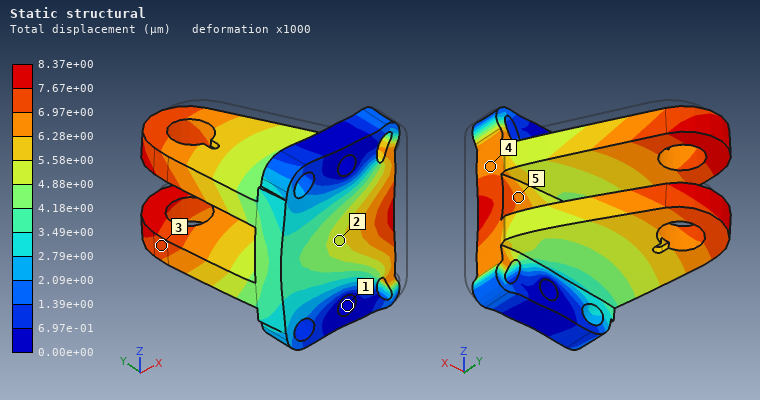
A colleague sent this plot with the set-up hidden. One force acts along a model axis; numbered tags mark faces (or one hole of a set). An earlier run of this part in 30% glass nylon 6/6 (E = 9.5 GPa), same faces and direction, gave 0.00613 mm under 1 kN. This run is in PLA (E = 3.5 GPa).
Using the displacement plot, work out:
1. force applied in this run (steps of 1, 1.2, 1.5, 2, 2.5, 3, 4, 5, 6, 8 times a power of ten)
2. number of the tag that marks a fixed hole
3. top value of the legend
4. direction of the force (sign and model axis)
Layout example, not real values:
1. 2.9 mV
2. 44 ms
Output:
1. 500 N
2. 1
3. 8.37e+00 µm
4. -X
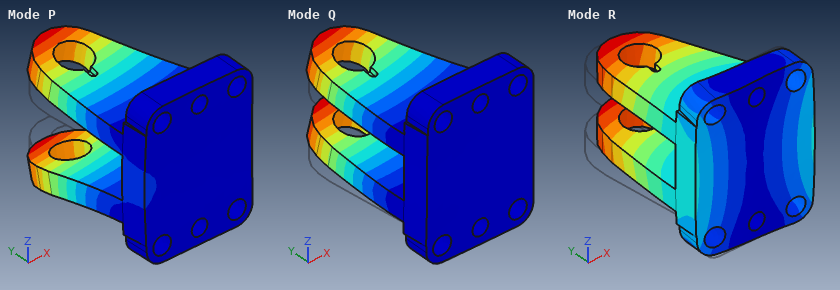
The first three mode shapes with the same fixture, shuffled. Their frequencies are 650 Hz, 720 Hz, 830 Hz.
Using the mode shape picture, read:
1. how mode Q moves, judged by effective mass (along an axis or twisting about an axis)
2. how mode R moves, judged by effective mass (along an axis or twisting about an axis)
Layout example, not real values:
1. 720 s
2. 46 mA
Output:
1. along Z
2. along X
